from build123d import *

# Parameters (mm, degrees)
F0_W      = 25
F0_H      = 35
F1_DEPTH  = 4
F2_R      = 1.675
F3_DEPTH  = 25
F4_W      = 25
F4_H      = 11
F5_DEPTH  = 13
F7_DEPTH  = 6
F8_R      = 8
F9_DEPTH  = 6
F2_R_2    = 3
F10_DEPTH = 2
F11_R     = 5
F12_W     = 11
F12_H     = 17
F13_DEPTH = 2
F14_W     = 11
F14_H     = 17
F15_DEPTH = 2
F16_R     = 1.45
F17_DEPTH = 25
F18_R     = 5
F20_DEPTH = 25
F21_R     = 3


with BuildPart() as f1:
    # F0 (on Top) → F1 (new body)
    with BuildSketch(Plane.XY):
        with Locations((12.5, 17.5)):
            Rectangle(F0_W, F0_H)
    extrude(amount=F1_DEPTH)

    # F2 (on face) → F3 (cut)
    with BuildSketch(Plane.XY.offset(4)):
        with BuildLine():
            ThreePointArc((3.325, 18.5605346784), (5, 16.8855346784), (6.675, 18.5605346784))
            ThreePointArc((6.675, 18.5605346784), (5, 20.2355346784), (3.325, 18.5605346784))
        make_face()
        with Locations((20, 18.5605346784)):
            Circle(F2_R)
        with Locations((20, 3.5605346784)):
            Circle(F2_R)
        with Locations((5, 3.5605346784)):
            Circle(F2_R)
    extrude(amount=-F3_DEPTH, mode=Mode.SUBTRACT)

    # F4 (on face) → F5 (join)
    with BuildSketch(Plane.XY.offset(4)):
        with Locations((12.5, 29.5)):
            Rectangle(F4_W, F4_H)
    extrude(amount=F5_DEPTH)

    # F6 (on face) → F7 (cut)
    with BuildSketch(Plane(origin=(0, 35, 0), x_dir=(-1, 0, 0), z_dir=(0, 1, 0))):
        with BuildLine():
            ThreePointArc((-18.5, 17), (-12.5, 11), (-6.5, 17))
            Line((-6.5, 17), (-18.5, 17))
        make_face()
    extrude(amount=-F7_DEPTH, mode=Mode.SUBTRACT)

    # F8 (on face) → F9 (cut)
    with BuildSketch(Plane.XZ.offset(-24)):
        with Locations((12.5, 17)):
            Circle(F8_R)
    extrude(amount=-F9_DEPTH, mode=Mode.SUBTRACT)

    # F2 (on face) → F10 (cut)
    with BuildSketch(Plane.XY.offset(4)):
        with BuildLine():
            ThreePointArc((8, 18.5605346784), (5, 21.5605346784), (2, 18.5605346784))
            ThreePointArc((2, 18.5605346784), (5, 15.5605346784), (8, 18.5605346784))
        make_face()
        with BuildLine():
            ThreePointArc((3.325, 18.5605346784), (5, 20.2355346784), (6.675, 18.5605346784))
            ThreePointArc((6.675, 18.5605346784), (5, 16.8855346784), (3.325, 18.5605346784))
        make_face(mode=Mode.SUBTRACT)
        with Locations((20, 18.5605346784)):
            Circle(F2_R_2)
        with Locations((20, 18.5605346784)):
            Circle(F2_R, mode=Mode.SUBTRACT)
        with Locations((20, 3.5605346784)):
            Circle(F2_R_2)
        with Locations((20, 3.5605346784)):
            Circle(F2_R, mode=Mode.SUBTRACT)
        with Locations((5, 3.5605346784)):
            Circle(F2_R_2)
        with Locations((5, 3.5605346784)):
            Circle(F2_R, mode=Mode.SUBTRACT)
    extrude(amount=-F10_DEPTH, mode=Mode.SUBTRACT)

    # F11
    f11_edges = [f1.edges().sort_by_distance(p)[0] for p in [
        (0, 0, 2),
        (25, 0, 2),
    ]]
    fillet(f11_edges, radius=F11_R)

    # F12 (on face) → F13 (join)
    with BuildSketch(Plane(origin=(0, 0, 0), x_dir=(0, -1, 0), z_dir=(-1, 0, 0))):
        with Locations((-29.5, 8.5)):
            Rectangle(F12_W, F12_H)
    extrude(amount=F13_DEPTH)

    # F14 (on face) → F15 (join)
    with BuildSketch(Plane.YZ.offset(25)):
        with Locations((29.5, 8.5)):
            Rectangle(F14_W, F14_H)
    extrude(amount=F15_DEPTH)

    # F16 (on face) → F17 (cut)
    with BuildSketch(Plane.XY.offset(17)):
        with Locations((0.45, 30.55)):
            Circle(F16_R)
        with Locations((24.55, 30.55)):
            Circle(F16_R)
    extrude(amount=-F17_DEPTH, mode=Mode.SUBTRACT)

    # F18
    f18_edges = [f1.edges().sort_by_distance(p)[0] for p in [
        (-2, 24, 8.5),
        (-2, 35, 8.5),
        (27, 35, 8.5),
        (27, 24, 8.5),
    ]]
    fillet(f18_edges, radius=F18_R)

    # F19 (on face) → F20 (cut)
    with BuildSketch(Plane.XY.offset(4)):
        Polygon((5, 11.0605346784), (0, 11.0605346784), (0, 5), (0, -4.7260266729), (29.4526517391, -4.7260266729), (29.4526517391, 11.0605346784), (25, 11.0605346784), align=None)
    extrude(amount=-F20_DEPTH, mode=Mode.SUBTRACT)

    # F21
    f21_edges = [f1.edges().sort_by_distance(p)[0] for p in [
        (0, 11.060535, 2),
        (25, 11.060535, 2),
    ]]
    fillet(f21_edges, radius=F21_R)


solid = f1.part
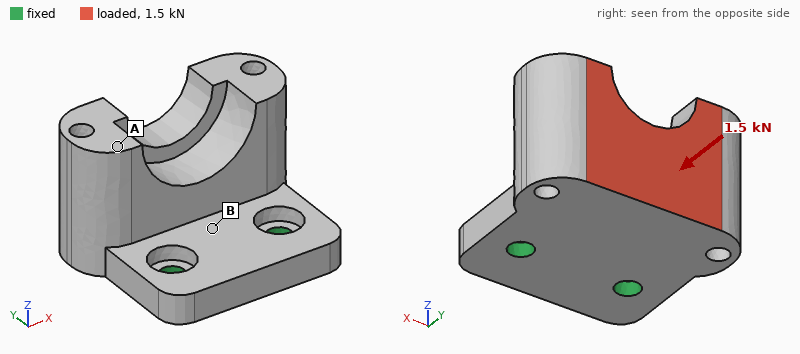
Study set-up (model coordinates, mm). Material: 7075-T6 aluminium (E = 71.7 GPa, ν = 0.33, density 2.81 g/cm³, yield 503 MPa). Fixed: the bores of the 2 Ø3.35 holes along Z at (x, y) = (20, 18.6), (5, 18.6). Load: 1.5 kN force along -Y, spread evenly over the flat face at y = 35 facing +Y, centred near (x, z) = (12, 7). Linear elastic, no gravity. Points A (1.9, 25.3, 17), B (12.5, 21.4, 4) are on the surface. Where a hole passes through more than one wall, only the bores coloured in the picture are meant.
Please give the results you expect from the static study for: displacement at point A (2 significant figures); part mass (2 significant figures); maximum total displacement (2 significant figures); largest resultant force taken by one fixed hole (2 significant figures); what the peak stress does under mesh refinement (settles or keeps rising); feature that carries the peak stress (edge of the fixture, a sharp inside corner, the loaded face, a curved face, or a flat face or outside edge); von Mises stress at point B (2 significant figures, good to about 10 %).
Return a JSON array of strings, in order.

["0.19 mm", "14 g", "0.24 mm", "750 N", "keeps rising", "edge of the fixture", "130 MPa"]
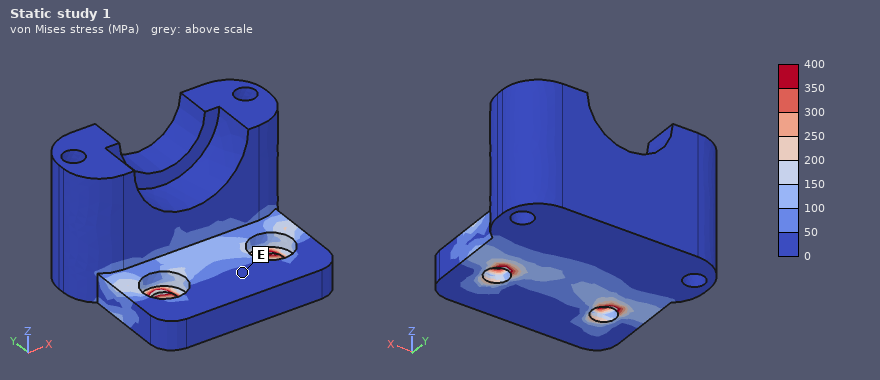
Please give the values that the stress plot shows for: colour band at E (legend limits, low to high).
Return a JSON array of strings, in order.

["0 to 50 MPa"]
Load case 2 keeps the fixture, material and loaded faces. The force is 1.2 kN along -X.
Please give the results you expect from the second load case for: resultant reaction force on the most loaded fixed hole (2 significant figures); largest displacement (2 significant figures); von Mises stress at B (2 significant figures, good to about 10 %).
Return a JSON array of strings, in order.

["1.4 kN", "26 µm", "34 MPa"]
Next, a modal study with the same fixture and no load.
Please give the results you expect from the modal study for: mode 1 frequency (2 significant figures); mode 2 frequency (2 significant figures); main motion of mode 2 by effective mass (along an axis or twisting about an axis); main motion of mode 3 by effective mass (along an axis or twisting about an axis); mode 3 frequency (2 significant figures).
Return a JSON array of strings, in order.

["3500 Hz", "9800 Hz", "along X", "along X", "16 kHz"]
